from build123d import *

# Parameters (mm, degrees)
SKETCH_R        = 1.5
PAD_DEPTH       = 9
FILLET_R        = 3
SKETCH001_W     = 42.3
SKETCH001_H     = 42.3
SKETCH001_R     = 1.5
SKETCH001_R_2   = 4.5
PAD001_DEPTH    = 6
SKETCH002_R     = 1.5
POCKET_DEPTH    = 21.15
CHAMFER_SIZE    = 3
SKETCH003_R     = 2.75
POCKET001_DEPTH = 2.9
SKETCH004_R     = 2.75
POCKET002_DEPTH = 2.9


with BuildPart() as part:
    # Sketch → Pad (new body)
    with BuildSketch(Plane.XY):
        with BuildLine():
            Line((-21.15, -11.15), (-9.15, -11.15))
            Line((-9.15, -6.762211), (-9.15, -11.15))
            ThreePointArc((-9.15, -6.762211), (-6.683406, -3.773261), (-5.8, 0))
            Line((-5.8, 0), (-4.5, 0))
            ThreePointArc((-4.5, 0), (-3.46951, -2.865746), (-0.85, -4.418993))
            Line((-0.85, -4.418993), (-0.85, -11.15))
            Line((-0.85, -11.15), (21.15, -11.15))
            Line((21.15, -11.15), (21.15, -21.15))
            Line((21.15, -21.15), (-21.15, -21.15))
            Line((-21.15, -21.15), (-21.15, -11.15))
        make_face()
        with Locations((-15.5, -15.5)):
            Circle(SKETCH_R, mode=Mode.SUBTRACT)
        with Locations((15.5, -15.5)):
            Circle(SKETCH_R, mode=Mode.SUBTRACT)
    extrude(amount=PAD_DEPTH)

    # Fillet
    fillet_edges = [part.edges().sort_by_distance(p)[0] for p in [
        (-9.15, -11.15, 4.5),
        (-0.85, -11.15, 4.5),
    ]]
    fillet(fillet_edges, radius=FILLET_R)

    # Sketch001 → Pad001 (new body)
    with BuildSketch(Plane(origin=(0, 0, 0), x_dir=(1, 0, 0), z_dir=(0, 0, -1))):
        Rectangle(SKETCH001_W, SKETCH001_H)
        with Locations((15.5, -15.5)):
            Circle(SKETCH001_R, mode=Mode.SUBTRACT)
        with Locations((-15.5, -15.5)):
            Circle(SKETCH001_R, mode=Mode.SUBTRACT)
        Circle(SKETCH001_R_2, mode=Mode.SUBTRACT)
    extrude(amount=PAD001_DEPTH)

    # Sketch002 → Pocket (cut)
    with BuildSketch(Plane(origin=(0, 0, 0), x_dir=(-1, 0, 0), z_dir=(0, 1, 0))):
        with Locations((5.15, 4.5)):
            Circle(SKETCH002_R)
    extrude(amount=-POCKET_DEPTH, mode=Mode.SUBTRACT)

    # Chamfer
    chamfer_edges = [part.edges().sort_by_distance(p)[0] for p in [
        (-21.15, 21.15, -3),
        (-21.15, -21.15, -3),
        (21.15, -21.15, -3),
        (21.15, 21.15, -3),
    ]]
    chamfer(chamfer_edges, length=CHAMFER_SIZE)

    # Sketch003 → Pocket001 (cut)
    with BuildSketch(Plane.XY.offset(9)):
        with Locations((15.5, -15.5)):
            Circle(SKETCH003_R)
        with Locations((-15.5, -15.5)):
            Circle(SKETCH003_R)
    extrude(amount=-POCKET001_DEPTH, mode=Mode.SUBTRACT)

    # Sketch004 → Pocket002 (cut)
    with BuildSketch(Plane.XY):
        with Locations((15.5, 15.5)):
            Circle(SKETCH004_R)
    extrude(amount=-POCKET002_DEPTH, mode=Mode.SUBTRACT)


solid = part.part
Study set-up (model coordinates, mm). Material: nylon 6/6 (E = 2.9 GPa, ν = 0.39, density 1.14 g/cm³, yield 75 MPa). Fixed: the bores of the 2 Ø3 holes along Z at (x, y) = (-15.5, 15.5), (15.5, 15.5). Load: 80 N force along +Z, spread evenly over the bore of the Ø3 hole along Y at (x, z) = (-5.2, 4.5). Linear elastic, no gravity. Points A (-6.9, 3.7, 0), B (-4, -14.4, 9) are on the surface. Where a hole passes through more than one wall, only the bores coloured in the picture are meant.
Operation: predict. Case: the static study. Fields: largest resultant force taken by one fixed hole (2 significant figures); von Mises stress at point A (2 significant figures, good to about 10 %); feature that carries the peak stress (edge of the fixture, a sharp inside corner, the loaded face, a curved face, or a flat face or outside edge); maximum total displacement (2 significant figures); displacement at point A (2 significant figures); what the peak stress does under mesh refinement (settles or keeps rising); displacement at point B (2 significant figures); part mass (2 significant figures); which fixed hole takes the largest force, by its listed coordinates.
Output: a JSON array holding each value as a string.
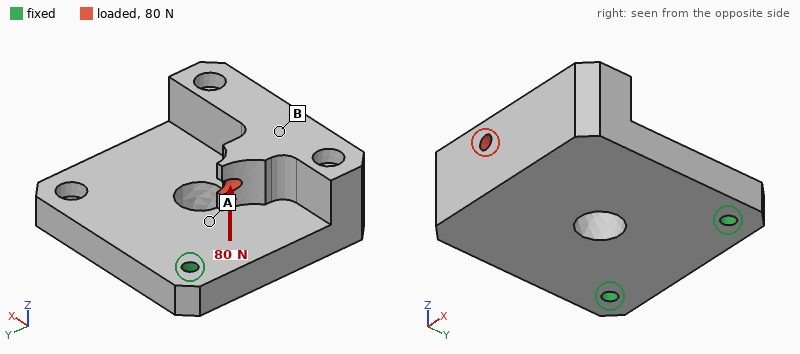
["58 N", "6.2 MPa", "edge of the fixture", "0.70 mm", "0.15 mm", "keeps rising", "0.56 mm", "16 g", "(-15.5, 15.5)"]
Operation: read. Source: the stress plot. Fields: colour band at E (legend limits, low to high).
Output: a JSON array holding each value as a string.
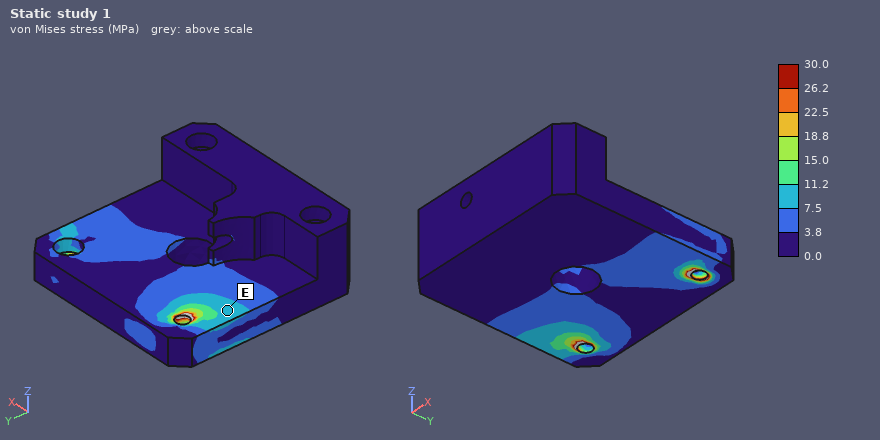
["7.5 to 11.2 MPa"]
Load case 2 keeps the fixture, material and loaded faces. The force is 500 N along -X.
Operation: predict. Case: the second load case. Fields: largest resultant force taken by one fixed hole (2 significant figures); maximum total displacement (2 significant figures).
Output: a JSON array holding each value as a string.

["520 N", "0.52 mm"]
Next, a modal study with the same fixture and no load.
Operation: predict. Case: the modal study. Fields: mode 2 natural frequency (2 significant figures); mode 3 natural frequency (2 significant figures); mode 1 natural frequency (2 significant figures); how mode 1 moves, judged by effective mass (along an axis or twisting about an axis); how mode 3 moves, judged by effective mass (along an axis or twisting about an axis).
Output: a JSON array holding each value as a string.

["1700 Hz", "2900 Hz", "580 Hz", "along Z", "along X"]
